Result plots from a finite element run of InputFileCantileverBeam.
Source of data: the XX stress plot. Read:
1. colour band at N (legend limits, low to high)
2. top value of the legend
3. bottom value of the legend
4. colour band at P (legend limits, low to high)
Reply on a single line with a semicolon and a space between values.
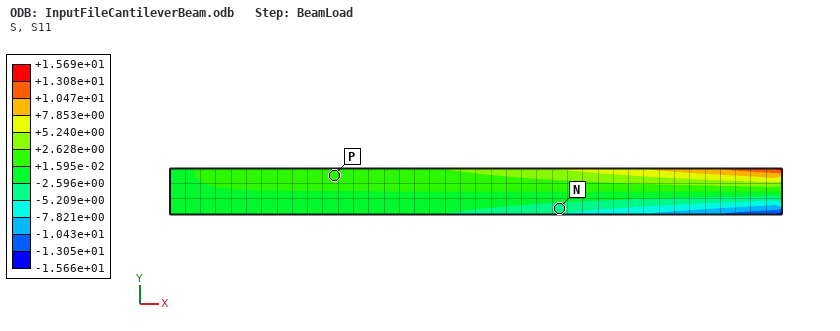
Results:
-5.209e+00 to -2.596e+00; +1.569e+01; -1.566e+01; +1.595e-02 to +2.628e+00
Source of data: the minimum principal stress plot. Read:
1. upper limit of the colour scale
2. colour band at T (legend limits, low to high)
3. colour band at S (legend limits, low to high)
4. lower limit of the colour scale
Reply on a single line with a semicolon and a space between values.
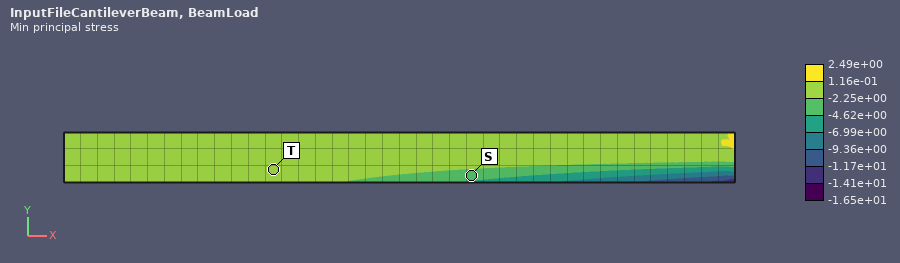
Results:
2.49e+00; -2.25e+00 to 1.16e-01; -4.62e+00 to -2.25e+00; -1.65e+01
